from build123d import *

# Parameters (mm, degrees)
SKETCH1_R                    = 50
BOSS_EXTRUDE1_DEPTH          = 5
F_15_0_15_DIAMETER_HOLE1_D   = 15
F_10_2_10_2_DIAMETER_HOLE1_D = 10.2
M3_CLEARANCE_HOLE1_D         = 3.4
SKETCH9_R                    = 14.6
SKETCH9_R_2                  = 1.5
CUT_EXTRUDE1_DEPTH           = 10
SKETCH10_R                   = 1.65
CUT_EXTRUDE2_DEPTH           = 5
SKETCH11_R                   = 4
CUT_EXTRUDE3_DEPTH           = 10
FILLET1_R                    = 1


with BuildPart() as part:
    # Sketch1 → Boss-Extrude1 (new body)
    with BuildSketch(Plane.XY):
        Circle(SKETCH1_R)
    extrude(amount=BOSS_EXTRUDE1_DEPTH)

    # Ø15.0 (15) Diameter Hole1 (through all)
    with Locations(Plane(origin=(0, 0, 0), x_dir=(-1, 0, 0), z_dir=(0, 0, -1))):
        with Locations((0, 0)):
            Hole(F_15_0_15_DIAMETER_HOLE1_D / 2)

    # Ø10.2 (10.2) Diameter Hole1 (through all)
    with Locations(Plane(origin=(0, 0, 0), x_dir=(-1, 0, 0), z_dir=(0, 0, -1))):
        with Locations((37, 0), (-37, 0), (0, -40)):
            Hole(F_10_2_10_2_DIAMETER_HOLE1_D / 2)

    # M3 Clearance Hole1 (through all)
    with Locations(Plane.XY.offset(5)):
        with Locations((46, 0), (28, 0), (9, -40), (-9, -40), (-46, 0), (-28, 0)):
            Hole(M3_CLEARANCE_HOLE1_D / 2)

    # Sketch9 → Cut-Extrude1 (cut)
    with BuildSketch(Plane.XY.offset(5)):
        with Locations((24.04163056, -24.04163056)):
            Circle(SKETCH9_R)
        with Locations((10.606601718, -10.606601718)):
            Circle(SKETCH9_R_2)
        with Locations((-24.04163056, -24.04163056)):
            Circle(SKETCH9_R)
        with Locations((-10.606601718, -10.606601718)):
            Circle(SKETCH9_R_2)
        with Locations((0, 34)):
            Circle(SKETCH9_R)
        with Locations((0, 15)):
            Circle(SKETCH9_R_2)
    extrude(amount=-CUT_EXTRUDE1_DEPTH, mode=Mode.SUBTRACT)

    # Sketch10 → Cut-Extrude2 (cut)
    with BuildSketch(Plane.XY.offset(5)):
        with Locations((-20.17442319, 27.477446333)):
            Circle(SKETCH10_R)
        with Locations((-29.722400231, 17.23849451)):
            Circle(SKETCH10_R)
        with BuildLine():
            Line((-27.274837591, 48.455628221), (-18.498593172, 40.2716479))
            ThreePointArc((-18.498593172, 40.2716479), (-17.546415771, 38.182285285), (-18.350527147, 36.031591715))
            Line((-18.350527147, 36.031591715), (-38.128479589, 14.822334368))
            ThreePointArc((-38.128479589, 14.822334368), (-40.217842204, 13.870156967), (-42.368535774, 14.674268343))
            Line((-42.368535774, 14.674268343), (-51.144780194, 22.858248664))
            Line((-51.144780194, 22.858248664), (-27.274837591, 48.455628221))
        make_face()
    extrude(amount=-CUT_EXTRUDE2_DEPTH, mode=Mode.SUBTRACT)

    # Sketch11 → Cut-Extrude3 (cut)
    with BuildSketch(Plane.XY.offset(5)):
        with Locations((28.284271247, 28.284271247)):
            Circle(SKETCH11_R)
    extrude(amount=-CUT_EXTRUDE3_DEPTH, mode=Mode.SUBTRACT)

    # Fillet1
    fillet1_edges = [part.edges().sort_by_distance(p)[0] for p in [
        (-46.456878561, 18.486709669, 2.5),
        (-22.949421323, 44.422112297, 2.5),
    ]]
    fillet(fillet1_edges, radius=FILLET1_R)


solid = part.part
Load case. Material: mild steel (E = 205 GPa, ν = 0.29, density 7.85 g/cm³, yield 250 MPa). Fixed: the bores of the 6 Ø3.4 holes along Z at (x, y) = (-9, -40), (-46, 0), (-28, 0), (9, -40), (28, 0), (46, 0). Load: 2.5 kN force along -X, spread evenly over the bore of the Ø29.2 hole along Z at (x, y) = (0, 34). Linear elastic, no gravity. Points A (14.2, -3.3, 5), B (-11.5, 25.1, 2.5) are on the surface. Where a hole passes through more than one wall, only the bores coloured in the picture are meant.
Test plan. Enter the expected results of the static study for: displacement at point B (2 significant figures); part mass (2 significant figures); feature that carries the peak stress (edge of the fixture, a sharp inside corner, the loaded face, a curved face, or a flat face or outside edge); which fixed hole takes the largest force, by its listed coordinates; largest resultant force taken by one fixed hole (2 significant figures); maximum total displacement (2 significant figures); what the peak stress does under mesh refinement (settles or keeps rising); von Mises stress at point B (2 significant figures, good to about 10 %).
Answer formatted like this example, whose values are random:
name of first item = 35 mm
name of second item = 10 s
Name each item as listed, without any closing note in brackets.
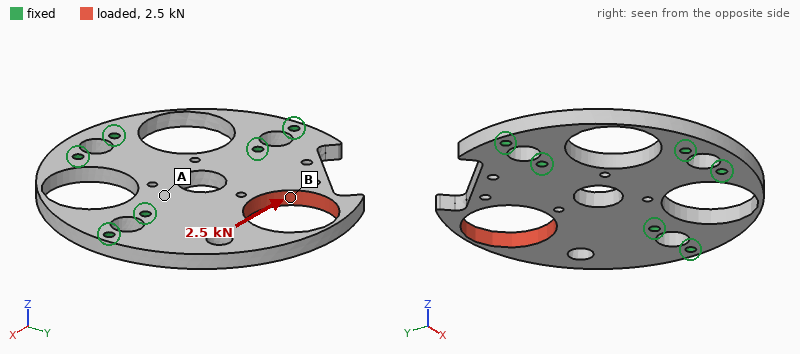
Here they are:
displacement at point B = 3.4 µm
part mass = 190 g
feature that carries the peak stress = a sharp inside corner
which fixed hole takes the largest force, by its listed coordinates = (46, 0)
largest resultant force taken by one fixed hole = 1.3 kN
maximum total displacement = 22 µm
what the peak stress does under mesh refinement = keeps rising
von Mises stress at point B = 41 MPa
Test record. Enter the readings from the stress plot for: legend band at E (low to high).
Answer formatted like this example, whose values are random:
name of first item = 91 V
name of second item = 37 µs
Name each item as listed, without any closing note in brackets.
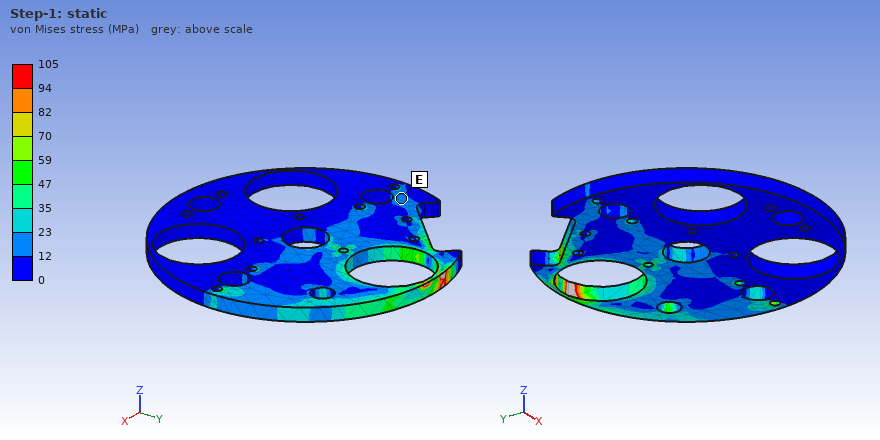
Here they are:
legend band at E = 12 to 23 MPa
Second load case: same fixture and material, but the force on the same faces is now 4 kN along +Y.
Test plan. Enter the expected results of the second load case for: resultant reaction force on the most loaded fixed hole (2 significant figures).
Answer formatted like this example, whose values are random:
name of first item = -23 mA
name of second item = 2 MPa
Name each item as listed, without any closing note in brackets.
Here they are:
resultant reaction force on the most loaded fixed hole = 1.6 kN
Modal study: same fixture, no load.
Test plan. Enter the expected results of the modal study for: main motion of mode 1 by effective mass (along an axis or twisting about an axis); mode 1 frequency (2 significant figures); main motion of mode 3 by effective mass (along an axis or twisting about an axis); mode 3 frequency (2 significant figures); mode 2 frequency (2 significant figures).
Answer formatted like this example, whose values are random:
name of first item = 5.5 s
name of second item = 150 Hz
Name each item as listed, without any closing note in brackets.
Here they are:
main motion of mode 1 by effective mass = along Z
mode 1 frequency = 2300 Hz
main motion of mode 3 by effective mass = along Z
mode 3 frequency = 7000 Hz
mode 2 frequency = 4200 Hz
